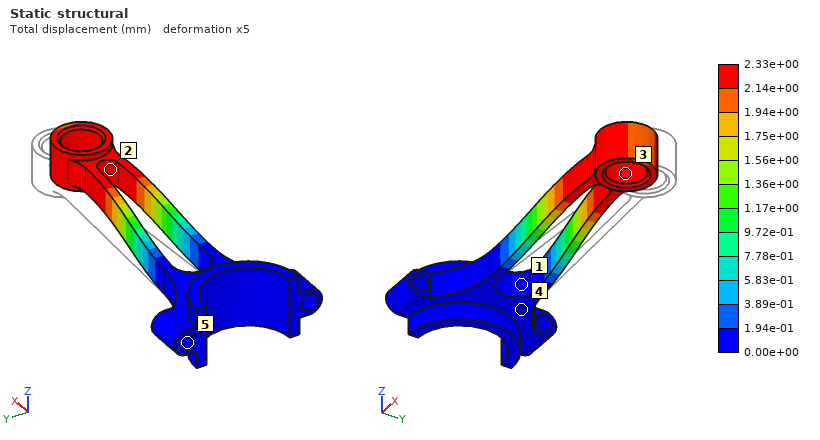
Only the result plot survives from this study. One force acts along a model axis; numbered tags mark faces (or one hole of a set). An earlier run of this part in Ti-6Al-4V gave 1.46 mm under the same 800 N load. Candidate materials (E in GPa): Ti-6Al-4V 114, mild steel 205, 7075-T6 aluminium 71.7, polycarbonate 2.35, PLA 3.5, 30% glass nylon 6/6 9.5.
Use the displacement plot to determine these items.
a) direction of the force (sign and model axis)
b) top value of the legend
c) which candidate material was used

-Y
2.33e+00 mm
7075-T6 aluminium
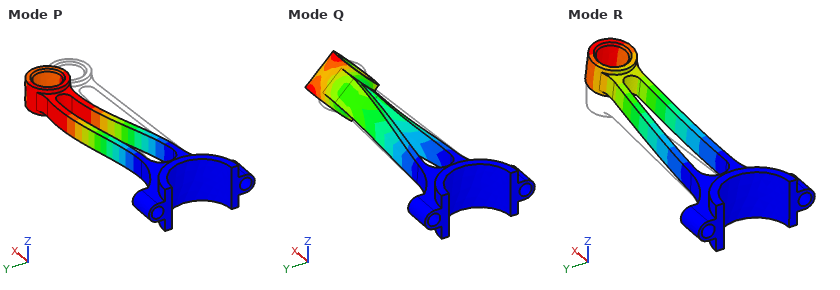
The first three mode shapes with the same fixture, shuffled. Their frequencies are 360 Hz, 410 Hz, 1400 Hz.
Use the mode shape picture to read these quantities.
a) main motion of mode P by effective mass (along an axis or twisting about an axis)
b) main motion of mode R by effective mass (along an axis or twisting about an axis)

along Y
along Z
